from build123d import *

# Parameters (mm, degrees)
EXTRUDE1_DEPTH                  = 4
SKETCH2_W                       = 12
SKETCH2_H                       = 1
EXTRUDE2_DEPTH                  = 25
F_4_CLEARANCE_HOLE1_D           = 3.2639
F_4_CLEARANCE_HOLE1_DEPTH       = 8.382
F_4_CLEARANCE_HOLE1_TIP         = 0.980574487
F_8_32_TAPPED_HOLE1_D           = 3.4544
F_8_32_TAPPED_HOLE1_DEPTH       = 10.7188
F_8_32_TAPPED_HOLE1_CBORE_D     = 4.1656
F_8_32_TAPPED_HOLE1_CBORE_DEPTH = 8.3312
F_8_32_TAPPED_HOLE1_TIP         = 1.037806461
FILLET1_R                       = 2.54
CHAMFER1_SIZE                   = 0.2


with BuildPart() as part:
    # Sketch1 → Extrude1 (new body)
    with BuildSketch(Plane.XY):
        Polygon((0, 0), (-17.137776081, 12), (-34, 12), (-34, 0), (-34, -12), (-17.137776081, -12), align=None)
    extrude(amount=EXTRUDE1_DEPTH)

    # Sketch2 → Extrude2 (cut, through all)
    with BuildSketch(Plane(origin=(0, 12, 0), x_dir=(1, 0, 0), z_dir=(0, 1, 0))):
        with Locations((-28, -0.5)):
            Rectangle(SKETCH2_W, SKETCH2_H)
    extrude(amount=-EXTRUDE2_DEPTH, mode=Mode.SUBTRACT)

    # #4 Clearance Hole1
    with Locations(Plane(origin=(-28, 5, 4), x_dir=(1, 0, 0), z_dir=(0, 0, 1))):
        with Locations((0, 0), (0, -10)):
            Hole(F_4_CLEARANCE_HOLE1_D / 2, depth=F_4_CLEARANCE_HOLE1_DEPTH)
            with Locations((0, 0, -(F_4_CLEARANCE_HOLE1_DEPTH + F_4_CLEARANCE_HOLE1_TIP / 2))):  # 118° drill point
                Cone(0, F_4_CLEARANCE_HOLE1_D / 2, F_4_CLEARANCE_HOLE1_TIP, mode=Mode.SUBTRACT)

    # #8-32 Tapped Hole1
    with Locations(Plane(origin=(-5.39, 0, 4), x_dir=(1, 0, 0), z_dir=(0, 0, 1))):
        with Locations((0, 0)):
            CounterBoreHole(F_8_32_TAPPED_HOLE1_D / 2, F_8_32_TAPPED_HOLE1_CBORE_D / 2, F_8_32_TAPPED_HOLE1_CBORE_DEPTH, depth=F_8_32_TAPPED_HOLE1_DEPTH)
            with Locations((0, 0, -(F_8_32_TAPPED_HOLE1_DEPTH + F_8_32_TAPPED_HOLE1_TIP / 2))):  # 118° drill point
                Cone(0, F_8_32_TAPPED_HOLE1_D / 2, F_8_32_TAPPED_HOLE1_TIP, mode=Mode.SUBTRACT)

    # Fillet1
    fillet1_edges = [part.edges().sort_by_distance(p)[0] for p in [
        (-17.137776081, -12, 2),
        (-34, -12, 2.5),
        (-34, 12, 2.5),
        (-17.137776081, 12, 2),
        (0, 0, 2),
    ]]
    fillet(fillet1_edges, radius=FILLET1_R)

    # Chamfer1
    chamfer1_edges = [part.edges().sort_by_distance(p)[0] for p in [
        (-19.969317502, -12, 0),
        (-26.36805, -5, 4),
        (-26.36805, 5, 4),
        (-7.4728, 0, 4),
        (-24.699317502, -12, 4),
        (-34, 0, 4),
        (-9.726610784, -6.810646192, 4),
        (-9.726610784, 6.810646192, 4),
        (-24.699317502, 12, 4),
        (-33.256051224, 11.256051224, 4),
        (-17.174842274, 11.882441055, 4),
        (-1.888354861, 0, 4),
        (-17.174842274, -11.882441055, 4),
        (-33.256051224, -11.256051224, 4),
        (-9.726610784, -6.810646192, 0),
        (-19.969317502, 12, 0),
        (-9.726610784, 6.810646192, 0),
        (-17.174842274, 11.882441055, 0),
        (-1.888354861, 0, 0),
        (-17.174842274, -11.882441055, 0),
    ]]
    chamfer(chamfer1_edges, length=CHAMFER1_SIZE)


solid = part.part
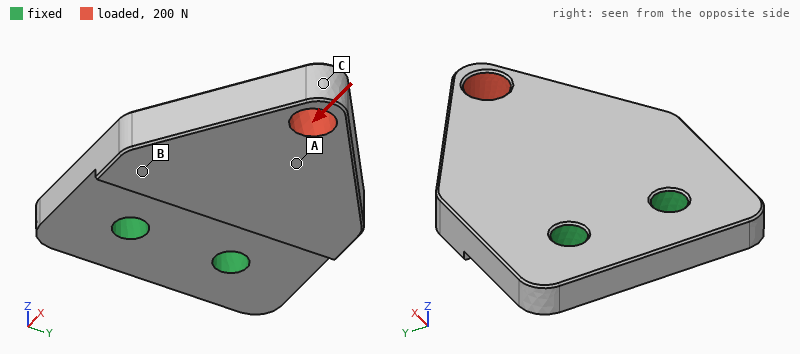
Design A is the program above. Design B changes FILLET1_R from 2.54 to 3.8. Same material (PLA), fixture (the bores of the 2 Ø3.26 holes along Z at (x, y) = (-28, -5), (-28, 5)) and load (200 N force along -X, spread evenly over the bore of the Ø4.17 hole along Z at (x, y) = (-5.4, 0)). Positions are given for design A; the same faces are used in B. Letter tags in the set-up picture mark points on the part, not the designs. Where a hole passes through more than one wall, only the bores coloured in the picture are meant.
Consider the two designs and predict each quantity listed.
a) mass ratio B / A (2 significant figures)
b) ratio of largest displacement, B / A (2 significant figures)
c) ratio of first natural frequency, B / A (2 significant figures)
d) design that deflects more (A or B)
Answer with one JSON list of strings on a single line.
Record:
["0.99", "1.1", "1.0", "B"]
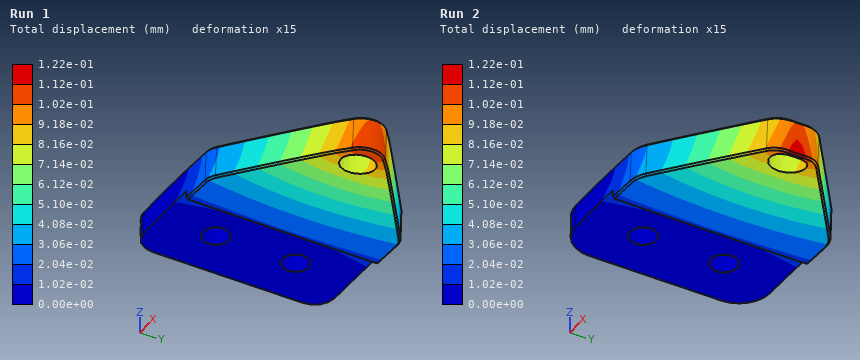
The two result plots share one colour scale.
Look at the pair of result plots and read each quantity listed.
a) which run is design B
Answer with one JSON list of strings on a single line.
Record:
["Run 2"]
